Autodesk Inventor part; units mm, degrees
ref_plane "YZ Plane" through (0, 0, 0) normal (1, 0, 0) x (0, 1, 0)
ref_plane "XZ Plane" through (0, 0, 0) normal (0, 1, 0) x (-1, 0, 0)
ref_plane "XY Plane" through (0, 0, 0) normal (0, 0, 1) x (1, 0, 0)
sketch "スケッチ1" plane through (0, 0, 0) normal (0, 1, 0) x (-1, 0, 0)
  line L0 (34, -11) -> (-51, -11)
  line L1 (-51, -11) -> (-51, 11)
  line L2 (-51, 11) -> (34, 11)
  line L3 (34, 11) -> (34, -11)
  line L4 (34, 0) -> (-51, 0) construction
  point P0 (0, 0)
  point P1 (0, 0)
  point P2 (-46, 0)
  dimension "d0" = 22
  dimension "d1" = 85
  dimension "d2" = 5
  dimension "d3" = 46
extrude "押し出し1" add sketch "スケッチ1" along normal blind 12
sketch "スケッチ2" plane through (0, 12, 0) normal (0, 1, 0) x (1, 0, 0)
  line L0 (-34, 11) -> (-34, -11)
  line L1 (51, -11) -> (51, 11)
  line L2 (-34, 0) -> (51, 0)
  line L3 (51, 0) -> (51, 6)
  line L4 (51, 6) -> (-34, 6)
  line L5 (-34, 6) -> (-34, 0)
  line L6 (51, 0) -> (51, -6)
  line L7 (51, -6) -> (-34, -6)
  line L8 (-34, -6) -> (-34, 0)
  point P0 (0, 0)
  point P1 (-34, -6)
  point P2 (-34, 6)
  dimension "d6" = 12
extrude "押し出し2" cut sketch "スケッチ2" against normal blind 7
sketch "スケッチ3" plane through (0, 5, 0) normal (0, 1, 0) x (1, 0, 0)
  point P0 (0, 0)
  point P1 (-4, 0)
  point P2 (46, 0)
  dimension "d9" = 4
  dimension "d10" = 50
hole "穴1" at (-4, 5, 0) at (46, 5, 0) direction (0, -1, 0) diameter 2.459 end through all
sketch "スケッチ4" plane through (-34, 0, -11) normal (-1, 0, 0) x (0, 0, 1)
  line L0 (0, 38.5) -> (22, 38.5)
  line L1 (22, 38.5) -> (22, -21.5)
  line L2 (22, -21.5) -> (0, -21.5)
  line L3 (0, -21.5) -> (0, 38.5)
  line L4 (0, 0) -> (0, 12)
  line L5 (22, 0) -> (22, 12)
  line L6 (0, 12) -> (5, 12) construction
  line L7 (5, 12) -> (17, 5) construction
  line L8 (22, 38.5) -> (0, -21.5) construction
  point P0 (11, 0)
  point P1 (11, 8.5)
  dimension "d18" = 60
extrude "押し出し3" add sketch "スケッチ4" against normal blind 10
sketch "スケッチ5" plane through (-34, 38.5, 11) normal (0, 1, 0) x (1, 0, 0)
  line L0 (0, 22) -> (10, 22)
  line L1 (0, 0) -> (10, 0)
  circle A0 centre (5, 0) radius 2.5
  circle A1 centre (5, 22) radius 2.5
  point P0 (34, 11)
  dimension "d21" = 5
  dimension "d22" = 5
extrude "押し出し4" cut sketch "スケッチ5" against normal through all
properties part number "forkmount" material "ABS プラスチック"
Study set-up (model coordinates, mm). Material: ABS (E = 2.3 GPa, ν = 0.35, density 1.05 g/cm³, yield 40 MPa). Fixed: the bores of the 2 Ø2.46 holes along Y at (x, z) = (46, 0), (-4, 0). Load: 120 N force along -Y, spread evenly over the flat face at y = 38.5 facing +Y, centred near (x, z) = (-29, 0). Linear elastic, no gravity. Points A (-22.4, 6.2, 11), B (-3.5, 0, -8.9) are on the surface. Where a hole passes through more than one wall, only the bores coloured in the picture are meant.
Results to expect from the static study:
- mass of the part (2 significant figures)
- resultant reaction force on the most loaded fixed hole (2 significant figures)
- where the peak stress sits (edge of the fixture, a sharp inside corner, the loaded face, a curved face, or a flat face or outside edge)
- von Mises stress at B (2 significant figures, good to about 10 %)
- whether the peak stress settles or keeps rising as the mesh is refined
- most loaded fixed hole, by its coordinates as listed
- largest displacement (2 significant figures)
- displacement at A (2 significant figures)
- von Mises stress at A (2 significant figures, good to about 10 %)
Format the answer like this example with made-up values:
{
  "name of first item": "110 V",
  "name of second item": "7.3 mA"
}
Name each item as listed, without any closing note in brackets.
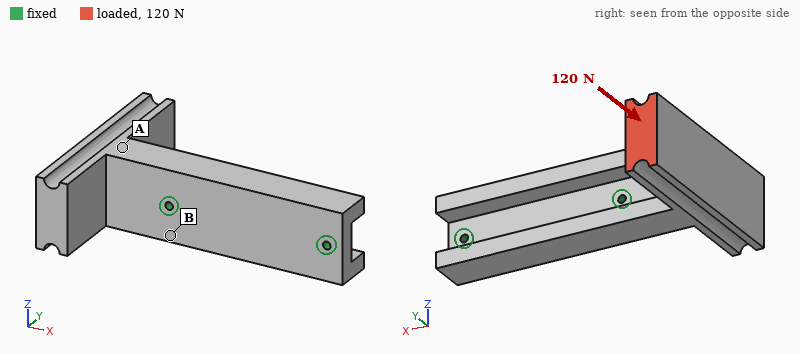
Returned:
{
  "mass of the part": "27 g",
  "resultant reaction force on the most loaded fixed hole": "190 N",
  "where the peak stress sits": "edge of the fixture",
  "von Mises stress at B": "5.4 MPa",
  "whether the peak stress settles or keeps rising as the mesh is refined": "keeps rising",
  "most loaded fixed hole, by its coordinates as listed": "(-4, 0)",
  "largest displacement": "0.69 mm",
  "displacement at A": "0.25 mm",
  "von Mises stress at A": "1.8 MPa"
}
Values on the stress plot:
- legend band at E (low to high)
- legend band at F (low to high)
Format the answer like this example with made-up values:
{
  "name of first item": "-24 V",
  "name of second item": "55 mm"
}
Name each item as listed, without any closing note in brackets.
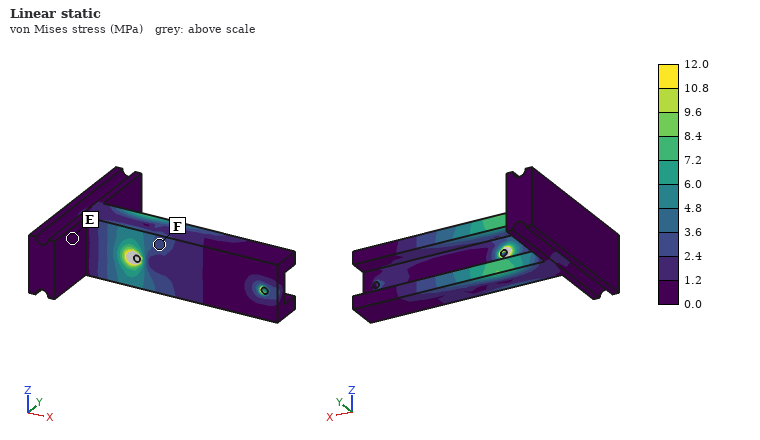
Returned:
{
  "legend band at E": "0.0 to 1.2 MPa",
  "legend band at F": "2.4 to 3.6 MPa"
}
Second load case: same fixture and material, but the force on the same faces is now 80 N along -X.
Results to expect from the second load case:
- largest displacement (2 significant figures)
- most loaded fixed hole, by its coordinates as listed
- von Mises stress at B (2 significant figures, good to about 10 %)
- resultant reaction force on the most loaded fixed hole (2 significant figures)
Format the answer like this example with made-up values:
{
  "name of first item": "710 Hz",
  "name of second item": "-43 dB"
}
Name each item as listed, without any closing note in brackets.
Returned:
{
  "largest displacement": "1.1 mm",
  "most loaded fixed hole, by its coordinates as listed": "(46, 0)",
  "von Mises stress at B": "4.7 MPa",
  "resultant reaction force on the most loaded fixed hole": "120 N"
}
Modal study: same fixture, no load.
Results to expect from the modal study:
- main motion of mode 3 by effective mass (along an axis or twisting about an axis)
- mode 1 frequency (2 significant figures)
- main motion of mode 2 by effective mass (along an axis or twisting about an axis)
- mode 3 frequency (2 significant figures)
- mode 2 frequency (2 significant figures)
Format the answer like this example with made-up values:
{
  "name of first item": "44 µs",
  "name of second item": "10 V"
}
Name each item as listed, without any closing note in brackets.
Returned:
{
  "main motion of mode 3 by effective mass": "along Z",
  "mode 1 frequency": "570 Hz",
  "main motion of mode 2 by effective mass": "along Y",
  "mode 3 frequency": "1300 Hz",
  "mode 2 frequency": "610 Hz"
}
